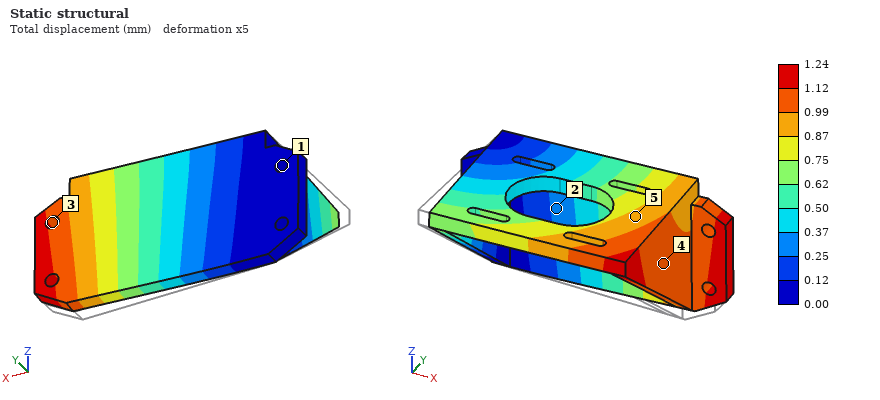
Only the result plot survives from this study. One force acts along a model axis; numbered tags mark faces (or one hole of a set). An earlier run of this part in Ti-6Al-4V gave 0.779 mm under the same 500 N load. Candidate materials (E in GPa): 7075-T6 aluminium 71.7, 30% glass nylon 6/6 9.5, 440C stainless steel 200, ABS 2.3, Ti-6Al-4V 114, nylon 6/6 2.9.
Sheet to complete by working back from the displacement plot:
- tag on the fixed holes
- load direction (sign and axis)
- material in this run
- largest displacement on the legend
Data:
1
+Y
7075-T6 aluminium
1.24 mm
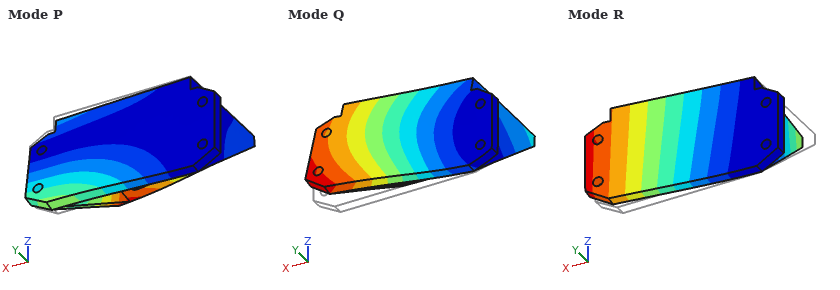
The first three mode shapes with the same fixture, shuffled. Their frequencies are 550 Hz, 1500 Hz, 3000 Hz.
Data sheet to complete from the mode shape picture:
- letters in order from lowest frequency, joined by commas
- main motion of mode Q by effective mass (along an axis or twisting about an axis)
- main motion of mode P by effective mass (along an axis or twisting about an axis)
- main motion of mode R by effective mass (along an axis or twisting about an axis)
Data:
R, P, Q
along Z
along Z
along Y
